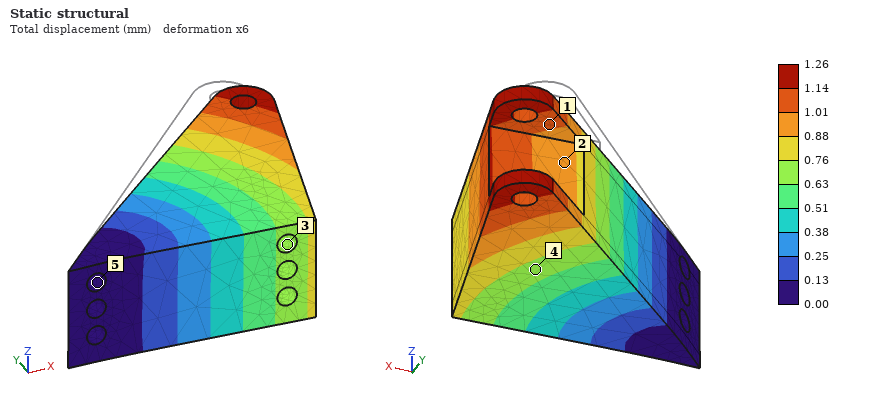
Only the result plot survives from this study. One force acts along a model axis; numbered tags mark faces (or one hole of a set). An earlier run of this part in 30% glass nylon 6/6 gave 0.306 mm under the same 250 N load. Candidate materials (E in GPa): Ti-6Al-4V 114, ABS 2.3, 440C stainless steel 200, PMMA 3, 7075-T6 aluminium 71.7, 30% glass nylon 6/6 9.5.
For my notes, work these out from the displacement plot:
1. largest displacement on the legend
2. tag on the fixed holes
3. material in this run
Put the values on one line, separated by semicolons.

1.26 mm; 5; ABS
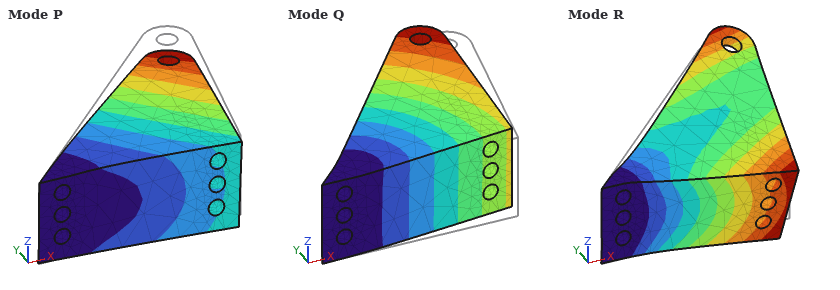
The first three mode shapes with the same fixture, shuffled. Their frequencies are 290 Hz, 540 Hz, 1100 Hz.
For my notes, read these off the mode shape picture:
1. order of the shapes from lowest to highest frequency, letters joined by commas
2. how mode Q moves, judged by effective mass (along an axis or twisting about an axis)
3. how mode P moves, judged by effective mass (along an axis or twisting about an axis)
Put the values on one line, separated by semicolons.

Q, P, R; along Y; along Z
